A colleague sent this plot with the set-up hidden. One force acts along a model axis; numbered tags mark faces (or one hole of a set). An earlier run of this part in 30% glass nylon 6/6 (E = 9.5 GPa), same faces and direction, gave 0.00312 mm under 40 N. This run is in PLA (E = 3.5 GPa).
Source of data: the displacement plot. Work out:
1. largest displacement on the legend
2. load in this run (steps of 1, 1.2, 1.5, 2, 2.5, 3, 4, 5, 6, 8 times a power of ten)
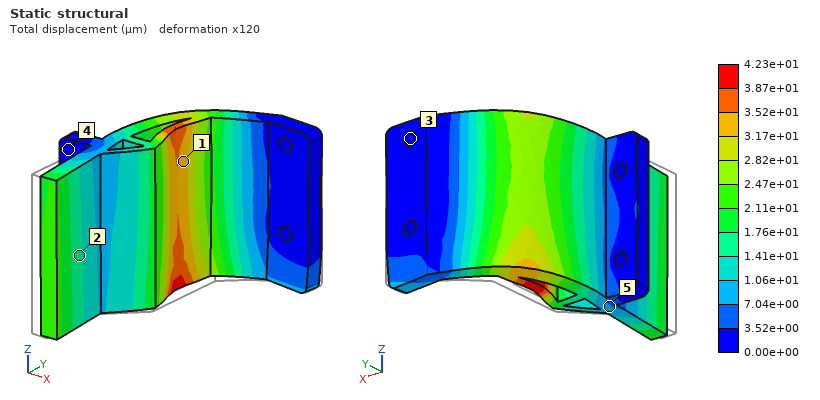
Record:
4.23e+01 µm
200 N
